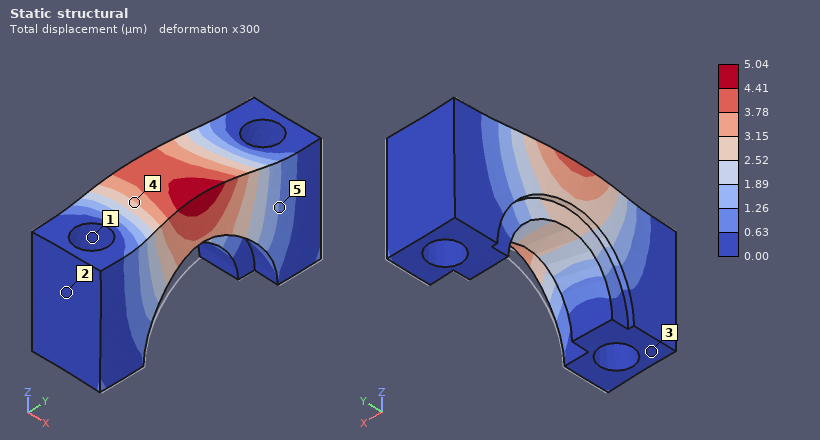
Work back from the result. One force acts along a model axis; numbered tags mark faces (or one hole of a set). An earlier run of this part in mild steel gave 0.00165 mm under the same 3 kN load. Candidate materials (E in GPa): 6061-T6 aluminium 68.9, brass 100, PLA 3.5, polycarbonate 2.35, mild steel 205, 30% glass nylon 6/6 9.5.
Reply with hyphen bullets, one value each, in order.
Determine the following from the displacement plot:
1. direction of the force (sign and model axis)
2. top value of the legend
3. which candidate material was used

- -X
- 5.04 µm
- 6061-T6 aluminium
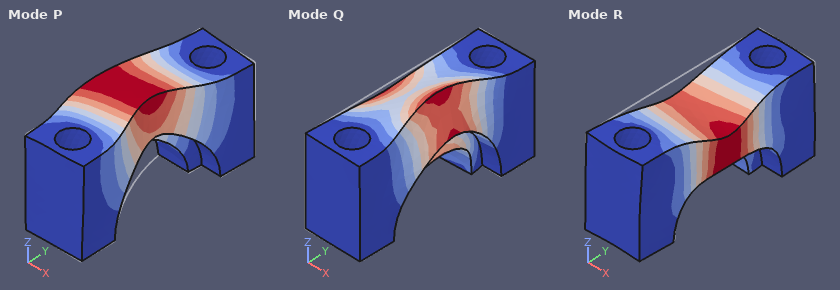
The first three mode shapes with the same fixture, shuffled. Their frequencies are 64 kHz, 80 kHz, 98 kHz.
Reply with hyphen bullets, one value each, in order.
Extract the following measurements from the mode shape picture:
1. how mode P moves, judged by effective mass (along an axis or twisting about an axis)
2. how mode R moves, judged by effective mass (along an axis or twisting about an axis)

- along X
- along Z
